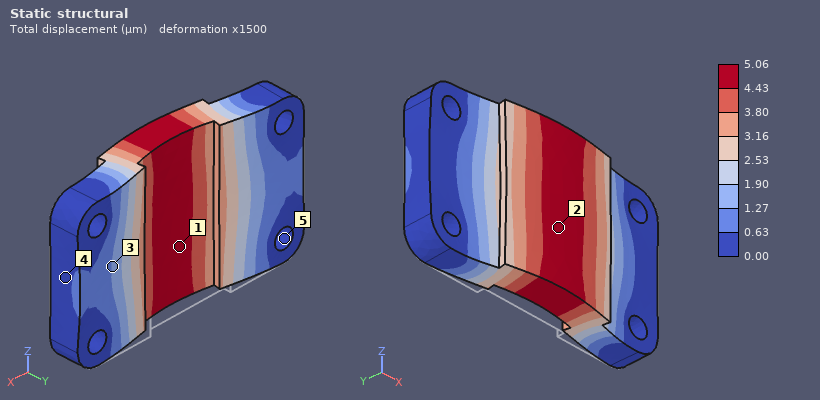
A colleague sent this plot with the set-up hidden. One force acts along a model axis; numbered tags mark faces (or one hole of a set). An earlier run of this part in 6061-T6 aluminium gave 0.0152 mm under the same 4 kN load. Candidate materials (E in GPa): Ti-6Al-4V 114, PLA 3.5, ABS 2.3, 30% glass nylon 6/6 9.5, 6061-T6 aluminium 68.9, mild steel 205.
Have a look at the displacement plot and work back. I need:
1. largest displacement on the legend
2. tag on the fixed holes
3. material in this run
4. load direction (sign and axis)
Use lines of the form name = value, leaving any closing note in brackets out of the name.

largest displacement on the legend = 5.06 µm
tag on the fixed holes = 5
material in this run = mild steel
load direction = -Y
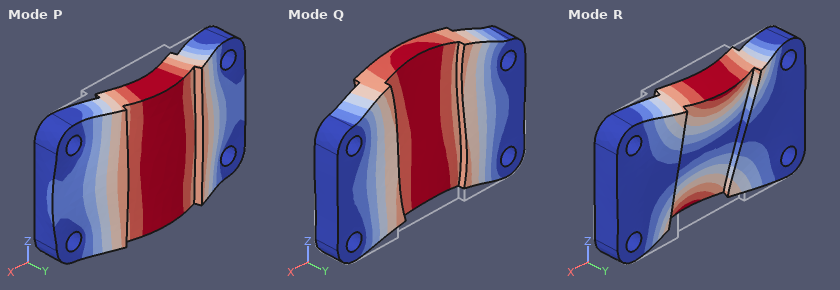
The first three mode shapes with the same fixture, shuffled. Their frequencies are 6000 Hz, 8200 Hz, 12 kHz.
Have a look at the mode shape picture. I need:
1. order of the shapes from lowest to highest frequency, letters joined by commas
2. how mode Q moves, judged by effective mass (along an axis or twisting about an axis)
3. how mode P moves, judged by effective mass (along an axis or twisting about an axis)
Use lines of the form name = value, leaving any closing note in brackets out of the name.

order of the shapes from lowest to highest frequency, letters joined by commas = P, R, Q
how mode Q moves, judged by effective mass = along Z
how mode P moves, judged by effective mass = along Y
